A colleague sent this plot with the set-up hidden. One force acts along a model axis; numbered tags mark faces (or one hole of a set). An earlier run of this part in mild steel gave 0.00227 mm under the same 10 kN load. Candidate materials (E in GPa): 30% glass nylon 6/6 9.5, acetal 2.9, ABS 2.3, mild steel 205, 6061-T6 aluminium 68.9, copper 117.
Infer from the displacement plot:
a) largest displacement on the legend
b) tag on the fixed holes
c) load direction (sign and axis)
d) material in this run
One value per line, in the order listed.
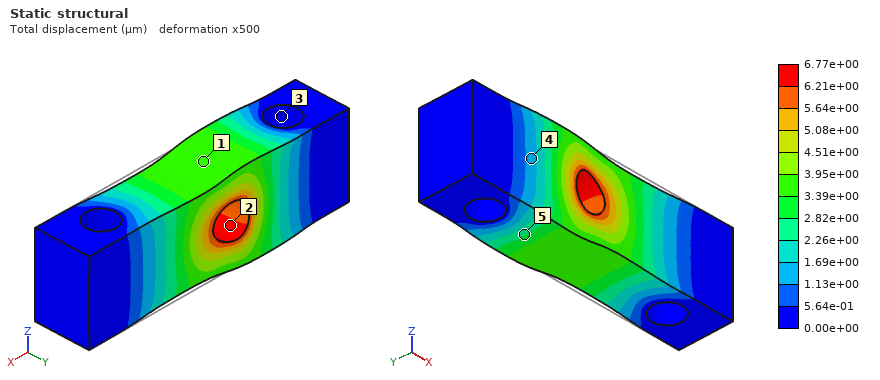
6.77e+00 µm
3
-X
6061-T6 aluminium
